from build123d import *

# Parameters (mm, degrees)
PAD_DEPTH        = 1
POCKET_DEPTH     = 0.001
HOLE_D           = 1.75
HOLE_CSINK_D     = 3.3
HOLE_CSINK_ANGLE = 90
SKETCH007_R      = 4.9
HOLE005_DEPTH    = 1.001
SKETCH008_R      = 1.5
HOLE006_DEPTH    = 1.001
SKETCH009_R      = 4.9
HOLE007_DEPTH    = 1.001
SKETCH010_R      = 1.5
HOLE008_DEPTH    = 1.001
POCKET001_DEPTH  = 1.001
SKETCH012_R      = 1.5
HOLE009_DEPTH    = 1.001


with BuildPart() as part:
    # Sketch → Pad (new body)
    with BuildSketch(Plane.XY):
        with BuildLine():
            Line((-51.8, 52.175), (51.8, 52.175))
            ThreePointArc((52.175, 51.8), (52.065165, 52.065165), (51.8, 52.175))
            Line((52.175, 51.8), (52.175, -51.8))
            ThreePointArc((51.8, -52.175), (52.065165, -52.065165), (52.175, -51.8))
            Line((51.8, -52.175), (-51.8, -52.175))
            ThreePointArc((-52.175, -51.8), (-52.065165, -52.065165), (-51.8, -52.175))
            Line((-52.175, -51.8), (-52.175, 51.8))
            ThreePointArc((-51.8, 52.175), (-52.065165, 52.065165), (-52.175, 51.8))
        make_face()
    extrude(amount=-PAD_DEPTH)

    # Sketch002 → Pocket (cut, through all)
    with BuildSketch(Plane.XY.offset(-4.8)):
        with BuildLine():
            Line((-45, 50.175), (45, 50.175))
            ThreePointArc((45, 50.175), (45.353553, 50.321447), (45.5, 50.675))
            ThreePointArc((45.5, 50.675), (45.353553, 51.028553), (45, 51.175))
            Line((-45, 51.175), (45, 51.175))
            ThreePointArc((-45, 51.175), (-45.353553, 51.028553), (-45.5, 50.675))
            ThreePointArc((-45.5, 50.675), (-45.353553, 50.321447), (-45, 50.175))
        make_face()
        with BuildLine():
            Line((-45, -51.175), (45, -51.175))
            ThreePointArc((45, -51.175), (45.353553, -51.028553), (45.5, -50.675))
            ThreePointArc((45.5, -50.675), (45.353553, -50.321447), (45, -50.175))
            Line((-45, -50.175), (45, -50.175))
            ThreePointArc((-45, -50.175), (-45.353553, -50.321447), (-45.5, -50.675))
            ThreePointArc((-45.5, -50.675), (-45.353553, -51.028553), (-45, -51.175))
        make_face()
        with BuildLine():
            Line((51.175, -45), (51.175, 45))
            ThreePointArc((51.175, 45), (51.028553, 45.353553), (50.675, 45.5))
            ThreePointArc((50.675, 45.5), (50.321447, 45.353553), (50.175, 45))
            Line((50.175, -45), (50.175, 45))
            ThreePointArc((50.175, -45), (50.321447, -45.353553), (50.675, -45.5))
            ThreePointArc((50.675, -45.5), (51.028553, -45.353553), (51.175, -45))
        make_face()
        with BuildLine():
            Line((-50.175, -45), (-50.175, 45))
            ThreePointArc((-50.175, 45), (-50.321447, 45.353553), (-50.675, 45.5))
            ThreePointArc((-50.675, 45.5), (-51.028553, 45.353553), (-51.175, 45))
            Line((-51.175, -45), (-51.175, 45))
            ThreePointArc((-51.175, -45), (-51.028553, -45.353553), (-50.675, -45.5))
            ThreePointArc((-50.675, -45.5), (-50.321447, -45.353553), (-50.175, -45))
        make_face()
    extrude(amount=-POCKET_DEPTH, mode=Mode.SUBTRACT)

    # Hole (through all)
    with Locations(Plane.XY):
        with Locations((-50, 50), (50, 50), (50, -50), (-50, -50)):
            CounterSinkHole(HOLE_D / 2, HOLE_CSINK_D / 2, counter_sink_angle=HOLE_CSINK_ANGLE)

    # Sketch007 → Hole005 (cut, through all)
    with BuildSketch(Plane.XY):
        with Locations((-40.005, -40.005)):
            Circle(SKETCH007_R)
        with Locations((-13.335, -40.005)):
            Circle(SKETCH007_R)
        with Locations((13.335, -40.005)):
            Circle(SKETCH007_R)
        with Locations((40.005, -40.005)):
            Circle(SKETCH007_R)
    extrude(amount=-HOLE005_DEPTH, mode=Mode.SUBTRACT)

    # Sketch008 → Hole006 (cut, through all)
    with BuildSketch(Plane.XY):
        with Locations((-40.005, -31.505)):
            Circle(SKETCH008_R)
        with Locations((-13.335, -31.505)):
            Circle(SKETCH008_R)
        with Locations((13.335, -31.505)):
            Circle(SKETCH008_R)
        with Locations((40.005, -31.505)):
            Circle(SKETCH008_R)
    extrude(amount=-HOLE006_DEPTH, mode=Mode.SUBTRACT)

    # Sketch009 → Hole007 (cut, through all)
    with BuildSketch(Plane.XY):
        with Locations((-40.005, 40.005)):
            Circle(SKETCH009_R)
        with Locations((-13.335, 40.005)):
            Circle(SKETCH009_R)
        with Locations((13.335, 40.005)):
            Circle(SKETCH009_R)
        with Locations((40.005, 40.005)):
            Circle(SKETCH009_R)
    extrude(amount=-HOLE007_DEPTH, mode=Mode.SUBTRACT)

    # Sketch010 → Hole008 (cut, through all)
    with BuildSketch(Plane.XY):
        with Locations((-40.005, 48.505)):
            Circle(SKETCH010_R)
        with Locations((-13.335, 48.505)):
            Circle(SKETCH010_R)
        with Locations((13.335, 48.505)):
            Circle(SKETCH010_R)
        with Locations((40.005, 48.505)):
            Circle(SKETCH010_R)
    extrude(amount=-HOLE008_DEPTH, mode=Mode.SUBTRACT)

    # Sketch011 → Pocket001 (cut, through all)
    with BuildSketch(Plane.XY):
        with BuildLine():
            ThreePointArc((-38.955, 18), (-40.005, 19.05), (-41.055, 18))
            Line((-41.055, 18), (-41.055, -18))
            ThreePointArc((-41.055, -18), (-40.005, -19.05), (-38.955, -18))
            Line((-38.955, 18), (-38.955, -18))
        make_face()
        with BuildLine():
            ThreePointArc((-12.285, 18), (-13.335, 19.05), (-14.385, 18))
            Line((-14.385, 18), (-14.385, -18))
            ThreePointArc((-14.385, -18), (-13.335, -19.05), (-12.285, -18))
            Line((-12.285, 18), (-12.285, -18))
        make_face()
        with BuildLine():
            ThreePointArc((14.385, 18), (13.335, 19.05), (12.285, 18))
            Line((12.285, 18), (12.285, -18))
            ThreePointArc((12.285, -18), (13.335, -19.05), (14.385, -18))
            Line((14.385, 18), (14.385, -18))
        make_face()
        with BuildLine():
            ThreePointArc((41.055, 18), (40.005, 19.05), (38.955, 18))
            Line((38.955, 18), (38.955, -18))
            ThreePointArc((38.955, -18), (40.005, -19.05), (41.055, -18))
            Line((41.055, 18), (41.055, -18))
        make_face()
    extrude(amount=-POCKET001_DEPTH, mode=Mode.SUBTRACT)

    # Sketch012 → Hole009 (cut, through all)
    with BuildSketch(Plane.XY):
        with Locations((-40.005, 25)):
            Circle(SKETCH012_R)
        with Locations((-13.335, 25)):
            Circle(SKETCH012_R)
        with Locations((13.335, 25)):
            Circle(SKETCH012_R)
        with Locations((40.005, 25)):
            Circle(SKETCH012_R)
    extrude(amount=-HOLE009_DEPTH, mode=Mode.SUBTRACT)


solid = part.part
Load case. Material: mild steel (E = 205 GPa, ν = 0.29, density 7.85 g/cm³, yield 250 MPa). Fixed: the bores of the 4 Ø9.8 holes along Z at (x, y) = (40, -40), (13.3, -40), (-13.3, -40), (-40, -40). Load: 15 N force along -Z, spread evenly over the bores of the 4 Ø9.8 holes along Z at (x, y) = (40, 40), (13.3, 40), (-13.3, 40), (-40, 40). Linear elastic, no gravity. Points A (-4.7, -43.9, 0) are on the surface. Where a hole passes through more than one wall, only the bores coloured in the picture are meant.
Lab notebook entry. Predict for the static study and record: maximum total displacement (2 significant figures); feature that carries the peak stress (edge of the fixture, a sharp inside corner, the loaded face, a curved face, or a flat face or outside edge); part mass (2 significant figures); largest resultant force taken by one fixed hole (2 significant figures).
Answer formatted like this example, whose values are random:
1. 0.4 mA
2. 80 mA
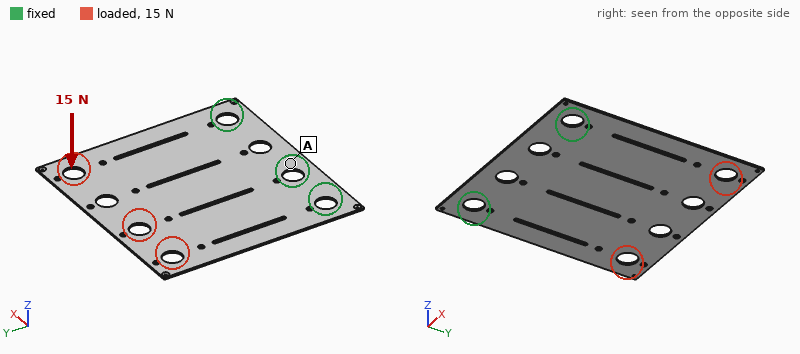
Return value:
1. 1.6 mm
2. a curved face
3. 77 g
4. 4.6 N
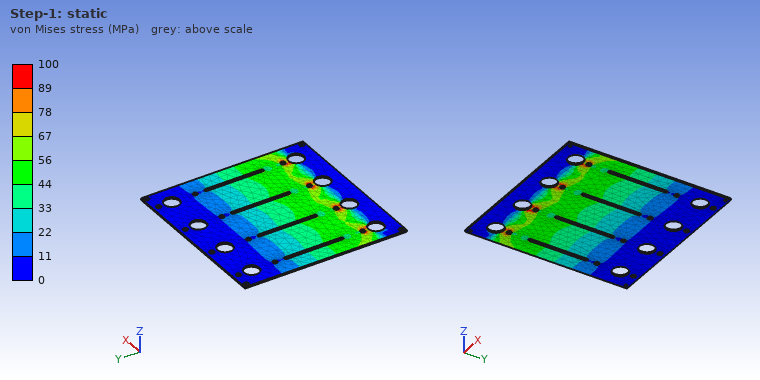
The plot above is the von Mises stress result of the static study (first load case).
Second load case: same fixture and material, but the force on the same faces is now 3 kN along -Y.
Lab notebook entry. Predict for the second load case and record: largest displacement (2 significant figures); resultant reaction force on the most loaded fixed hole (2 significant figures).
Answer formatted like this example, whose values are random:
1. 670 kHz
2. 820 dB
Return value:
1. 14 µm
2. 780 N
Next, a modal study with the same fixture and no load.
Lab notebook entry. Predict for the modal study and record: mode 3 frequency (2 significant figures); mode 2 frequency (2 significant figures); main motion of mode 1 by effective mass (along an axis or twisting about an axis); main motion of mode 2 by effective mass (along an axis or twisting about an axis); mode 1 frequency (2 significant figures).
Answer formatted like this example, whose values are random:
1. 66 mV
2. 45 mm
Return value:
1. 580 Hz
2. 240 Hz
3. along Z
4. twisting about Y
5. 110 Hz
